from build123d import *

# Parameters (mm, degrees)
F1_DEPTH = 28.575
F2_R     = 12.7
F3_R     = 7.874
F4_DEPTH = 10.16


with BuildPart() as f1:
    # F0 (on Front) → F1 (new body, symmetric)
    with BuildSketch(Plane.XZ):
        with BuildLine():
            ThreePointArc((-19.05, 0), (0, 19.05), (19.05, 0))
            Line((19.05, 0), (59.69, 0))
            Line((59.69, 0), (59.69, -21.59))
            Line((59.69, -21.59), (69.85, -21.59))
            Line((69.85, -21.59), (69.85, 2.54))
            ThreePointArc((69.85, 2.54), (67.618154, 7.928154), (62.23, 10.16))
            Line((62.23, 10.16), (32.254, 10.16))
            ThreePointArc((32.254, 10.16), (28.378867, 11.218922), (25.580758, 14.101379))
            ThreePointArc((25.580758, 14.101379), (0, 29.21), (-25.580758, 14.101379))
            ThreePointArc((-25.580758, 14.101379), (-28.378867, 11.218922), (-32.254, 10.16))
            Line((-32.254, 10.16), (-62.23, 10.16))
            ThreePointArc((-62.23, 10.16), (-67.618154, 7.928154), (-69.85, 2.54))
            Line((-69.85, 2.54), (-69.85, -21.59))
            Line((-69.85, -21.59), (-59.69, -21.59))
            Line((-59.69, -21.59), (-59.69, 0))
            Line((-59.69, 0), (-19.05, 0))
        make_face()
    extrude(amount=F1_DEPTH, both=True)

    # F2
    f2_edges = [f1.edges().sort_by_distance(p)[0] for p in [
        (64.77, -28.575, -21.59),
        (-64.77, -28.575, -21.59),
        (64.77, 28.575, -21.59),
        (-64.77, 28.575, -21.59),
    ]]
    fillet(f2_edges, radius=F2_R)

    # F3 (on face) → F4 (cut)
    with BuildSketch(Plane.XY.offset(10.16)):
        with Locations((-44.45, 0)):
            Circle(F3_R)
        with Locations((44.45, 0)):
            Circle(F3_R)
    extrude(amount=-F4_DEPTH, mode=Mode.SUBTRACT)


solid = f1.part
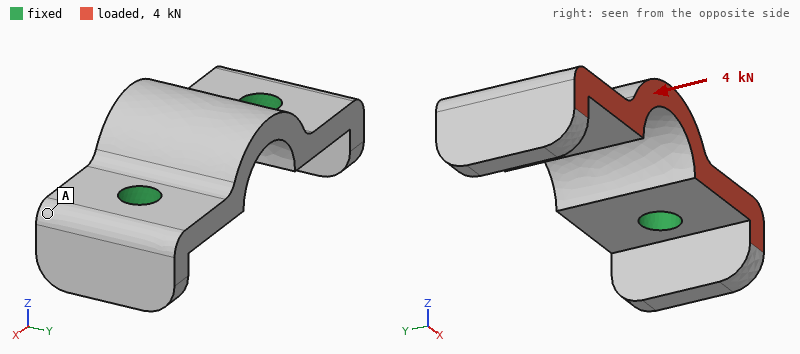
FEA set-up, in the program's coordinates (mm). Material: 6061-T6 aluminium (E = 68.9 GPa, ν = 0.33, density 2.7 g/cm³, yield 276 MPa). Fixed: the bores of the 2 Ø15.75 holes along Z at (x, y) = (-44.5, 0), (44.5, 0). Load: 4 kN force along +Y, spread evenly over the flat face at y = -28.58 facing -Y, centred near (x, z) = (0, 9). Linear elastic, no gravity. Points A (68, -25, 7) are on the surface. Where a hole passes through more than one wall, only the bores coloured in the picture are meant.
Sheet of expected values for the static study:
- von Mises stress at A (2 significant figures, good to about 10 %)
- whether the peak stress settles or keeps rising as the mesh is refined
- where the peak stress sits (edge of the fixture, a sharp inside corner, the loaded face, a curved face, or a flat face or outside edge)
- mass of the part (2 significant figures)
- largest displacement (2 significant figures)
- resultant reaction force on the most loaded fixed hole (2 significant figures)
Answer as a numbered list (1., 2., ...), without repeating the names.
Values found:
1. 2.1 MPa
2. keeps rising
3. edge of the fixture
4. 300 g
5. 13 µm
6. 2.0 kN
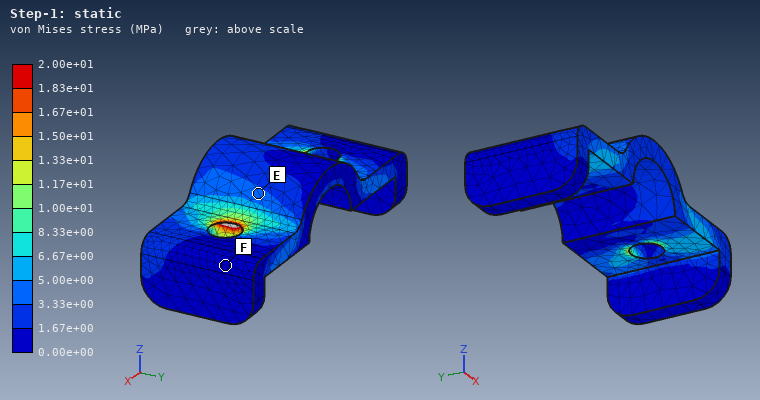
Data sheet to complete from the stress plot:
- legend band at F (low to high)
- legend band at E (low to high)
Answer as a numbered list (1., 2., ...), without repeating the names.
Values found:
1. 0.00e+00 to 1.67e+00 MPa
2. 3.33e+00 to 5.00e+00 MPa
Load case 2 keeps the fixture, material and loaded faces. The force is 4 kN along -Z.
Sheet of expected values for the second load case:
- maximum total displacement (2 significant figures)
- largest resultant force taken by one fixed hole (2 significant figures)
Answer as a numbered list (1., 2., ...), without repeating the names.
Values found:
1. 41 µm
2. 2.1 kN
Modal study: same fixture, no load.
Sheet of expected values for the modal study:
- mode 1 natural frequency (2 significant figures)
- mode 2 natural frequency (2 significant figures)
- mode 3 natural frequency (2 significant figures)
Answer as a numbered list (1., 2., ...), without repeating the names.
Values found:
1. 5300 Hz
2. 5900 Hz
3. 5900 Hz
